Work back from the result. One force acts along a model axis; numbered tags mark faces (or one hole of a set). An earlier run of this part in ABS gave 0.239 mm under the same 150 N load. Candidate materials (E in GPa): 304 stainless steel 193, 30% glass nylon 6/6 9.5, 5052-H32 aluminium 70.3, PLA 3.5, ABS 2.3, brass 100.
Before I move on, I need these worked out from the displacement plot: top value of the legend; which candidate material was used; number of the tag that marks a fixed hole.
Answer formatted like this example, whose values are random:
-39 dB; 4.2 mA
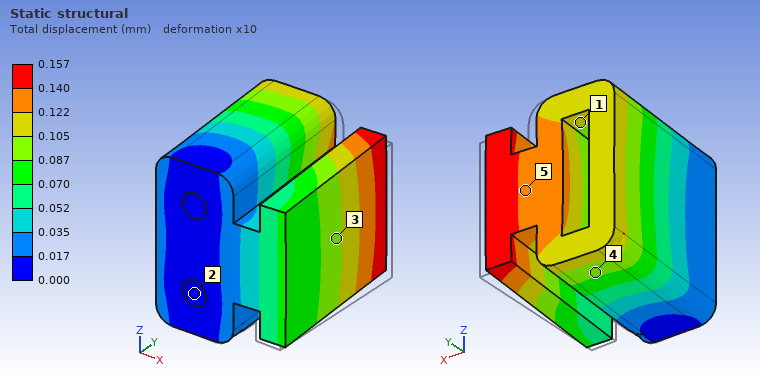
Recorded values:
0.157 mm; PLA; 2
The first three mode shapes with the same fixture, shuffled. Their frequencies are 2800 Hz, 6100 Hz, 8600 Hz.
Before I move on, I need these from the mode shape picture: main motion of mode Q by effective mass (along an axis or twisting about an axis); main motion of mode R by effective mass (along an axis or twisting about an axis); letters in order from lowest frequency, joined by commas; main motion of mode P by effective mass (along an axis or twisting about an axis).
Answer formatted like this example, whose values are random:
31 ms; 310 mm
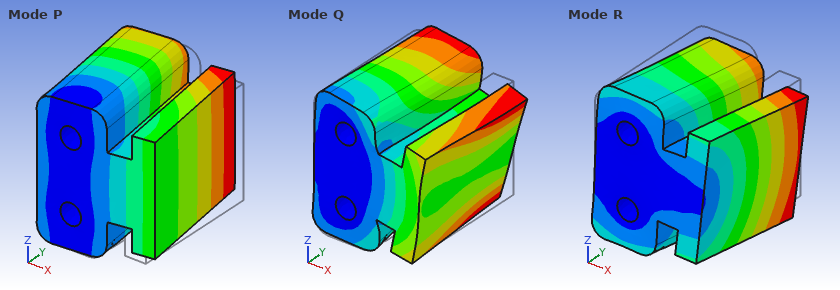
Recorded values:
twisting about Y; along Z; P, R, Q; along X
